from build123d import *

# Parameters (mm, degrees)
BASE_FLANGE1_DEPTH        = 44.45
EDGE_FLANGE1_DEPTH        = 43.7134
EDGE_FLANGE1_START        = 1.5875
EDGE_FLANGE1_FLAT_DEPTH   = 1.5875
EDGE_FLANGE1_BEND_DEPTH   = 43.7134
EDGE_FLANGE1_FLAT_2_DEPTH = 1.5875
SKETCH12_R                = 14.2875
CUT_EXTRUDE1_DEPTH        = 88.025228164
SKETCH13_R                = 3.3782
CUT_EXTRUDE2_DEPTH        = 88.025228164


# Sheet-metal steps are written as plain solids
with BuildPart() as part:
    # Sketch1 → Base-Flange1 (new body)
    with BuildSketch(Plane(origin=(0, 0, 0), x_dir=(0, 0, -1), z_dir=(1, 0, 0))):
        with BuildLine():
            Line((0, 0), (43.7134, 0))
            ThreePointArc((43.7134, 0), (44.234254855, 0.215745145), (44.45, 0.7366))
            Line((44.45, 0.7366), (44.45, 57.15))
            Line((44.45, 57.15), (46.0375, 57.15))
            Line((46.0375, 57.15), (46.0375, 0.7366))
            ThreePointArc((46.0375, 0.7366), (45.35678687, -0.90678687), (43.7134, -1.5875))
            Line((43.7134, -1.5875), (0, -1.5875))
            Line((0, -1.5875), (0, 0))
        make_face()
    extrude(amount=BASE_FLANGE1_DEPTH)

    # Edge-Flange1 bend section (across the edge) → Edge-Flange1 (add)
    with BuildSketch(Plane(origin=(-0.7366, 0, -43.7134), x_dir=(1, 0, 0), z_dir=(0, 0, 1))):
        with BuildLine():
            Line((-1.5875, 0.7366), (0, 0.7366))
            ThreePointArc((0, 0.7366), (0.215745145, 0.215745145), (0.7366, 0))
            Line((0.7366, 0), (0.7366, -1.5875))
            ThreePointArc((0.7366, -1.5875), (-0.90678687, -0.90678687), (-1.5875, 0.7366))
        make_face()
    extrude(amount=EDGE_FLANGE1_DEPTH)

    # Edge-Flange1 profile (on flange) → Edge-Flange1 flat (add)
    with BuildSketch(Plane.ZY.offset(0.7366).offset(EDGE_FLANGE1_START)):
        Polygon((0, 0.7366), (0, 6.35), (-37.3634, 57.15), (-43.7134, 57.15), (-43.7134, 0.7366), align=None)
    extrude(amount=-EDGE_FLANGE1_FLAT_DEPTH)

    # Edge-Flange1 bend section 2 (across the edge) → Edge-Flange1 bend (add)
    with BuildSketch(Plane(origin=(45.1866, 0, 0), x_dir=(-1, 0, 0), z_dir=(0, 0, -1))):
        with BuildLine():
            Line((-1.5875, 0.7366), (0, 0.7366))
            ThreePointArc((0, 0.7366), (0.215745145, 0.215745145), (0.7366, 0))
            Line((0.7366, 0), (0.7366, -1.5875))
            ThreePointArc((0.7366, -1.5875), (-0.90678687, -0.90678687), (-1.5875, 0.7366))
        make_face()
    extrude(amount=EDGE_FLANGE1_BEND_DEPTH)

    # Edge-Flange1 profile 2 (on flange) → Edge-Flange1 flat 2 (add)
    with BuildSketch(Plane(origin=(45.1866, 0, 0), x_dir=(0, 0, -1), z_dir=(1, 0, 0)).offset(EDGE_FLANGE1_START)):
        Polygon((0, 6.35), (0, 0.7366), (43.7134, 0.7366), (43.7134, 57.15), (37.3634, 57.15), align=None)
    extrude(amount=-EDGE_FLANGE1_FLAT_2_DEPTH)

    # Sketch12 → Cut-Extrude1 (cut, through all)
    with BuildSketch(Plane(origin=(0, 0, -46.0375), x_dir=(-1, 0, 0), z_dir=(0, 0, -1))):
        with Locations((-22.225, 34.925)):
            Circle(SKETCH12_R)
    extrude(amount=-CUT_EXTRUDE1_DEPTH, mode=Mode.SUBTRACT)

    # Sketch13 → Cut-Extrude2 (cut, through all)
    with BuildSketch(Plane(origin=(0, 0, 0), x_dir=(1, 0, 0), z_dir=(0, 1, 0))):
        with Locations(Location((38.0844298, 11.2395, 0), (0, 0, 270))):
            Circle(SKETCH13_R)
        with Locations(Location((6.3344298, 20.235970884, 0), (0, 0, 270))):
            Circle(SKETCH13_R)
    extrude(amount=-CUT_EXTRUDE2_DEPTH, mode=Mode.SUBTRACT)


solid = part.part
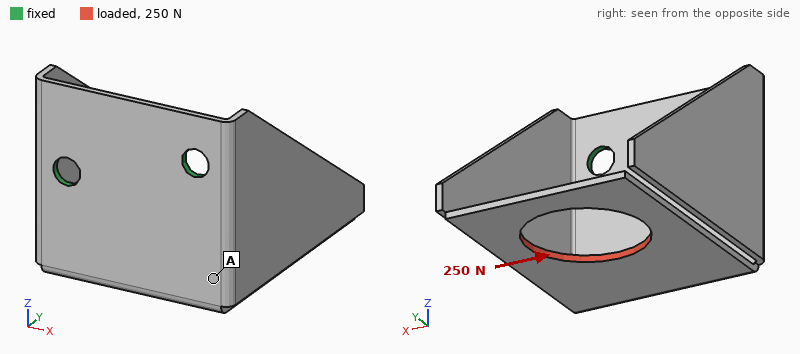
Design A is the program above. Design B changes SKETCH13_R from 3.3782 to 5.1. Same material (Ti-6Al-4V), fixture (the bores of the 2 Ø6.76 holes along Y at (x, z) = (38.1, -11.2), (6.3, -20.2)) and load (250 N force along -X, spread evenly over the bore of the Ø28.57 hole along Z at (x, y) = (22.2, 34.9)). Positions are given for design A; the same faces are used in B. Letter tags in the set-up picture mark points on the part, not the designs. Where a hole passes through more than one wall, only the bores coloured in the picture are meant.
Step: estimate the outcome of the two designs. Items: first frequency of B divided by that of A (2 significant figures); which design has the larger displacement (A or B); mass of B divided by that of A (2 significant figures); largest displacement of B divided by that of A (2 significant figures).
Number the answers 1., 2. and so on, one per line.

1. 1.0
2. A
3. 0.99
4. 0.59
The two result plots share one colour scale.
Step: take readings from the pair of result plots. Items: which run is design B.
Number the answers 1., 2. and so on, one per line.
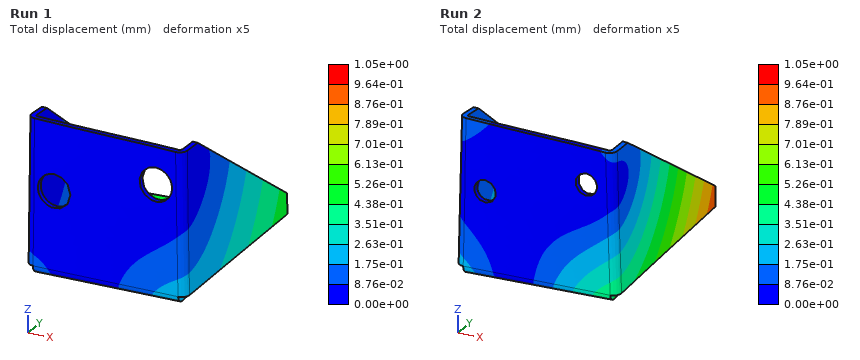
1. Run 1
